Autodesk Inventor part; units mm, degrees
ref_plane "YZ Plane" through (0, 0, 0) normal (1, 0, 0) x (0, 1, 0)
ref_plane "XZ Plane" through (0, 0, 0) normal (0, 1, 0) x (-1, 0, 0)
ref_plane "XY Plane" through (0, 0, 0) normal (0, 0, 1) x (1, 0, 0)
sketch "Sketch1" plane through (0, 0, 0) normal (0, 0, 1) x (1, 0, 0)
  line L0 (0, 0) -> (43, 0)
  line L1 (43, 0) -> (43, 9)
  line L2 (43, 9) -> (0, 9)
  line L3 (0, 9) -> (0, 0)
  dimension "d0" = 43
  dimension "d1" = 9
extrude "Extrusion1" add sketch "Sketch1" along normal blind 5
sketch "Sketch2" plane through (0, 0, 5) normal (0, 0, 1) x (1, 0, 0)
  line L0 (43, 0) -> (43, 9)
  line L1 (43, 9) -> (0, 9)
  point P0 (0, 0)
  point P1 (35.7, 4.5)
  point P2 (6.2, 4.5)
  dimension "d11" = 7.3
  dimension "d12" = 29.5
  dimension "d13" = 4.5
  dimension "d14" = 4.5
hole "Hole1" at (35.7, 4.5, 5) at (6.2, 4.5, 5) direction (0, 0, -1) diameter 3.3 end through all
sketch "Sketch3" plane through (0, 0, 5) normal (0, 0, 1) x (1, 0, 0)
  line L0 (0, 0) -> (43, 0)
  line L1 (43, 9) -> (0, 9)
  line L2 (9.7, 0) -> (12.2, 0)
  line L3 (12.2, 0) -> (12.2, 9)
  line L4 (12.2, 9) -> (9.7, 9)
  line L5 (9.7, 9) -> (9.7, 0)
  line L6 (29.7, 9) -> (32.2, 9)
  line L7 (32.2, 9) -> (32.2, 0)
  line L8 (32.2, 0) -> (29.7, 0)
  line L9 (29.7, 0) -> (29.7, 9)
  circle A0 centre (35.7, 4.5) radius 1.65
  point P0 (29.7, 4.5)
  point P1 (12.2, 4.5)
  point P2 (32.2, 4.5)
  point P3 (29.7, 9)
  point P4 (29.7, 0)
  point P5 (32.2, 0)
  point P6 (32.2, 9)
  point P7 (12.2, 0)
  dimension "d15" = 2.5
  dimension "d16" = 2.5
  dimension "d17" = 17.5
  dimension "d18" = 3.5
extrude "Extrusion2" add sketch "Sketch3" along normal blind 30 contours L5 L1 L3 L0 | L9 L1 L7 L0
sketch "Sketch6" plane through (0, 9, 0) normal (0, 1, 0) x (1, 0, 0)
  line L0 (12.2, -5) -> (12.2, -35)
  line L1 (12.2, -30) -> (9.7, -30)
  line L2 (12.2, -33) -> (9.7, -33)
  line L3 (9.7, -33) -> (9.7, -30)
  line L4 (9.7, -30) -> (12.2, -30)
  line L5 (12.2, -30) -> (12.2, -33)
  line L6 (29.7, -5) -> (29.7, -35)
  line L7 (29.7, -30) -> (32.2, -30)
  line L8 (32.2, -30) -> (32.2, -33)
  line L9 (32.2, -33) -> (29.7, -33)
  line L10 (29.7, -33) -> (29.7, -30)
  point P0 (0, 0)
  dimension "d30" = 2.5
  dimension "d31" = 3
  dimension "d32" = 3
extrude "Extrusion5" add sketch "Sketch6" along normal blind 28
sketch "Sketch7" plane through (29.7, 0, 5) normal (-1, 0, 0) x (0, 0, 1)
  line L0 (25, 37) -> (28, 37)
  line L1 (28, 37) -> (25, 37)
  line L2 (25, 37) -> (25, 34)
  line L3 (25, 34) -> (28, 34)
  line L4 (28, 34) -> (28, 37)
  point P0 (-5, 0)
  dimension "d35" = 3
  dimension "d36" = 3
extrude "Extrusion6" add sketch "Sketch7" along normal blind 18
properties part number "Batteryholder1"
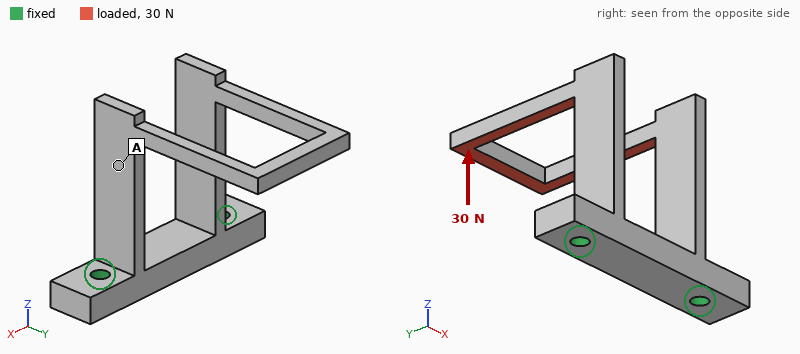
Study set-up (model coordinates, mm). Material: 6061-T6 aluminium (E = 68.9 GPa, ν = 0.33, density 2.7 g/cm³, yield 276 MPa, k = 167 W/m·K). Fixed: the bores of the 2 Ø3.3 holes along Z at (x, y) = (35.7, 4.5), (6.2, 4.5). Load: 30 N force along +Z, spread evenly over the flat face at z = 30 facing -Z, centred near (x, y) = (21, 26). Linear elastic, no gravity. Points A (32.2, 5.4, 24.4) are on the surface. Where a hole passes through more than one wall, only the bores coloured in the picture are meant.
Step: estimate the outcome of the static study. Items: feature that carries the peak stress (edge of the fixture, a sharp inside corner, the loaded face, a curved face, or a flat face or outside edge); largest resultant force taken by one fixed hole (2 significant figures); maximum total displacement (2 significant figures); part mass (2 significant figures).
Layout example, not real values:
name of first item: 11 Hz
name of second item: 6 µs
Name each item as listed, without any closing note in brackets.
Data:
feature that carries the peak stress: a flat face or outside edge
largest resultant force taken by one fixed hole: 15 N
maximum total displacement: 0.21 mm
part mass: 10 g
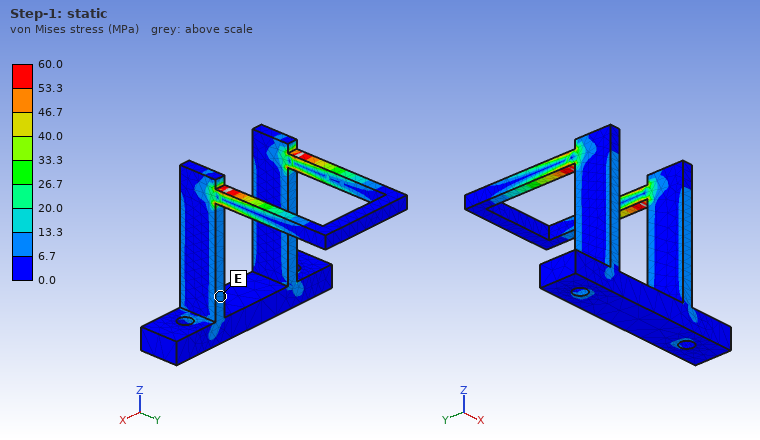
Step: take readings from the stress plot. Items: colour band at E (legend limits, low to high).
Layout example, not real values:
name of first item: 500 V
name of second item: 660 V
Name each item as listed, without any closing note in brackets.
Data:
colour band at E: 6.7 to 13.3 MPa
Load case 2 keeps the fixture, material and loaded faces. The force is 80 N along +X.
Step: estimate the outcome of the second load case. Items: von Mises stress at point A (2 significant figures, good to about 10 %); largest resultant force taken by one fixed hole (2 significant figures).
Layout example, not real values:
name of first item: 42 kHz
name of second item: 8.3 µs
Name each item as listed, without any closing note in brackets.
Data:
von Mises stress at point A: 62 MPa
largest resultant force taken by one fixed hole: 95 N
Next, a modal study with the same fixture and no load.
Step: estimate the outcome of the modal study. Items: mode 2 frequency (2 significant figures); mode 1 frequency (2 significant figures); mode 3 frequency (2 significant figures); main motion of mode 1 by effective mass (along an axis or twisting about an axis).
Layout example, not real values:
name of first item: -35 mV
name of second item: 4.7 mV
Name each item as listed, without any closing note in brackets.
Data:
mode 2 frequency: 1700 Hz
mode 1 frequency: 1300 Hz
mode 3 frequency: 2400 Hz
main motion of mode 1 by effective mass: along X
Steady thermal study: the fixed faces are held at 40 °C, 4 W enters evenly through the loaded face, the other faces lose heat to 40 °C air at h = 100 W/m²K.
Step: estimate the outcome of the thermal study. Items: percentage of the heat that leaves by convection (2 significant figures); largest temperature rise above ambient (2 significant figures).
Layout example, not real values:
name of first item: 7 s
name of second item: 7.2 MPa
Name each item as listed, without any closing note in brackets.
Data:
percentage of the heat that leaves by convection: 52 %
largest temperature rise above ambient: 28 K
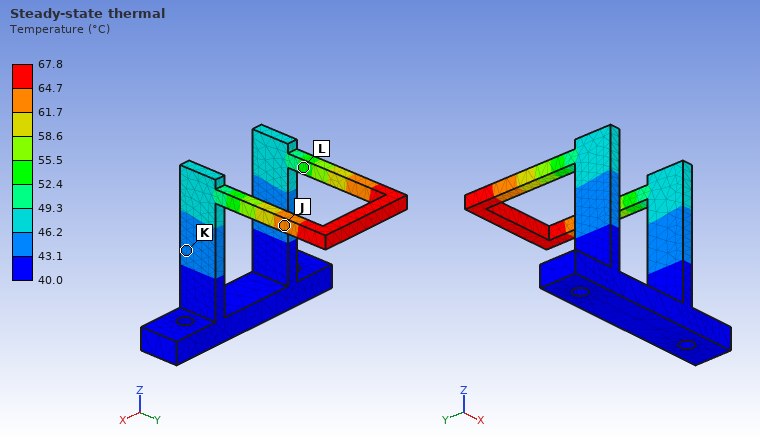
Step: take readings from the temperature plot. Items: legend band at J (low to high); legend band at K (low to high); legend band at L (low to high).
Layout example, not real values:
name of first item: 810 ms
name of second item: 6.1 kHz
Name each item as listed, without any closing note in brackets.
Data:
legend band at J: 61.7 to 64.7 °C
legend band at K: 43.1 to 46.2 °C
legend band at L: 52.4 to 55.5 °C
